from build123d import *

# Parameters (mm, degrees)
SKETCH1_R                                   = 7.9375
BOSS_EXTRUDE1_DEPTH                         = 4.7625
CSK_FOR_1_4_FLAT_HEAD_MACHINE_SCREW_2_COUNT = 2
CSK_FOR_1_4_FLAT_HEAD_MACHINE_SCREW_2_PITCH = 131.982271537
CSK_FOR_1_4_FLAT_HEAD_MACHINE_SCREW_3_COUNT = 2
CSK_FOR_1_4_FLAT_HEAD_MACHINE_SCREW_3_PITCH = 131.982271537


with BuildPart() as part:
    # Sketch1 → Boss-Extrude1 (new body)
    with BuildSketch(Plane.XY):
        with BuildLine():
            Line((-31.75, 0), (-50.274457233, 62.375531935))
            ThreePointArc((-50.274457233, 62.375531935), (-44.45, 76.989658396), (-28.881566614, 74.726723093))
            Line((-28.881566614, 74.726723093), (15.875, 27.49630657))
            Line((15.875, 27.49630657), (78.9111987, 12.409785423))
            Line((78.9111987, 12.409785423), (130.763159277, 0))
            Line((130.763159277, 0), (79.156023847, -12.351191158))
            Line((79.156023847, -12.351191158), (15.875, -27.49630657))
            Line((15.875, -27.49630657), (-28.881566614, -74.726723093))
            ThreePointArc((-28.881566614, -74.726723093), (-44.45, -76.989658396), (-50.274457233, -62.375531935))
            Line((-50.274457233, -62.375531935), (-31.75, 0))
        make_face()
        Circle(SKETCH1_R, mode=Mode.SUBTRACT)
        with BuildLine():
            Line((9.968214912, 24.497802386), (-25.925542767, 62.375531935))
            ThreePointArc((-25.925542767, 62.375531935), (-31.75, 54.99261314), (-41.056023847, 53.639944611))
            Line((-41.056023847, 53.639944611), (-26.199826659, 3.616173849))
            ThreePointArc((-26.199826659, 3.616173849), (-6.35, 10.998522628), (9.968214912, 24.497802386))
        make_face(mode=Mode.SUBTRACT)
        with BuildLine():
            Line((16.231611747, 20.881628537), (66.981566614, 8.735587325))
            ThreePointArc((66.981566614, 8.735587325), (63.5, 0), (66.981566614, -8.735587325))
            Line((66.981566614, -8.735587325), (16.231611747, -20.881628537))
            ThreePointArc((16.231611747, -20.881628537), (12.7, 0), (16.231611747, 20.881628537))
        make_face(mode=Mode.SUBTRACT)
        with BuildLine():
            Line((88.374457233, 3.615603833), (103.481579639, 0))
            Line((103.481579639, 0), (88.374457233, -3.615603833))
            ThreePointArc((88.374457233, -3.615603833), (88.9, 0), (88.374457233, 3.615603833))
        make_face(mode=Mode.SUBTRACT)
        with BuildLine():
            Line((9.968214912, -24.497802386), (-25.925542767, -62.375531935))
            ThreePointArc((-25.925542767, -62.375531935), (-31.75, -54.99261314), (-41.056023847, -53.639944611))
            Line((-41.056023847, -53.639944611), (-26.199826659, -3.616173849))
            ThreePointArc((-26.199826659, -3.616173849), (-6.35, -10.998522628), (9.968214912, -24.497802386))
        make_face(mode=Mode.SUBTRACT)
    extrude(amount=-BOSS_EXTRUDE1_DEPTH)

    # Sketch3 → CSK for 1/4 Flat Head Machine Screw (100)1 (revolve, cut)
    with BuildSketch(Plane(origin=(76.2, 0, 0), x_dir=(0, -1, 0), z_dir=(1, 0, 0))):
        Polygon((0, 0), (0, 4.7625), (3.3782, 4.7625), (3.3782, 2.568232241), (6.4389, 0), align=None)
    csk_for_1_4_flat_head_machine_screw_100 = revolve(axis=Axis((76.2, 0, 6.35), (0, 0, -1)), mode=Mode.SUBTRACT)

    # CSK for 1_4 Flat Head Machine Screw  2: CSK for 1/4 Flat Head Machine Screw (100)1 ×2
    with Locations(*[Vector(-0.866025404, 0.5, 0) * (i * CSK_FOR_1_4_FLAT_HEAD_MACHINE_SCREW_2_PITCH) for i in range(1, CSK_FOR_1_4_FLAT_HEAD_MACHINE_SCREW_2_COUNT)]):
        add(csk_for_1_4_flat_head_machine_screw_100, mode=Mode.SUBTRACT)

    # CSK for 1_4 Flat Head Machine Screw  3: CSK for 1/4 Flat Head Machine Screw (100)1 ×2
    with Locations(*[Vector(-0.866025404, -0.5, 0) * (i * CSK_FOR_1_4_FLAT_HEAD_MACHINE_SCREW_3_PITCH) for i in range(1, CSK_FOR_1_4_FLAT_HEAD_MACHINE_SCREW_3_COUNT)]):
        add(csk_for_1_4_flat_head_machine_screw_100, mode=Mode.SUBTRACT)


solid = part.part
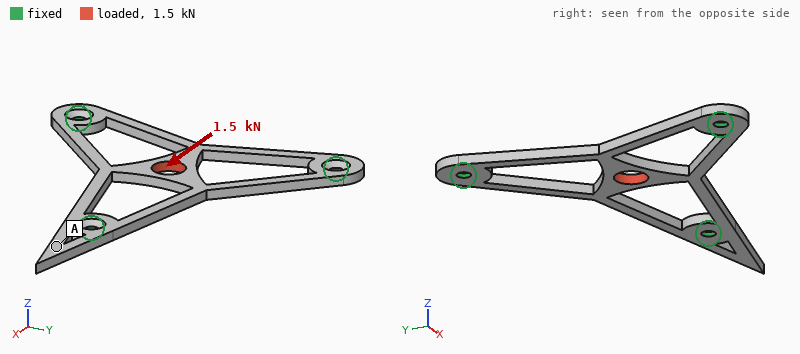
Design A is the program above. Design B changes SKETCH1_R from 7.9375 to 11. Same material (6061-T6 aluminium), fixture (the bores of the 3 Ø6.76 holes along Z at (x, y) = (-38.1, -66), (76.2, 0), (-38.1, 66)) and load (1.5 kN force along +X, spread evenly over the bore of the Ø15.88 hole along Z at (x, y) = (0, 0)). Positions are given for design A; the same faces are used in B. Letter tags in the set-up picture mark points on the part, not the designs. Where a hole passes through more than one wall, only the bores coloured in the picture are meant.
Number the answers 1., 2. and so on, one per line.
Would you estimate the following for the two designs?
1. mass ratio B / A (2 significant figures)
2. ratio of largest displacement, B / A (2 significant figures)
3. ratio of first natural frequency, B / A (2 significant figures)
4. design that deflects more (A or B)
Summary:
1. 0.96
2. 2.0
3. 1.0
4. B
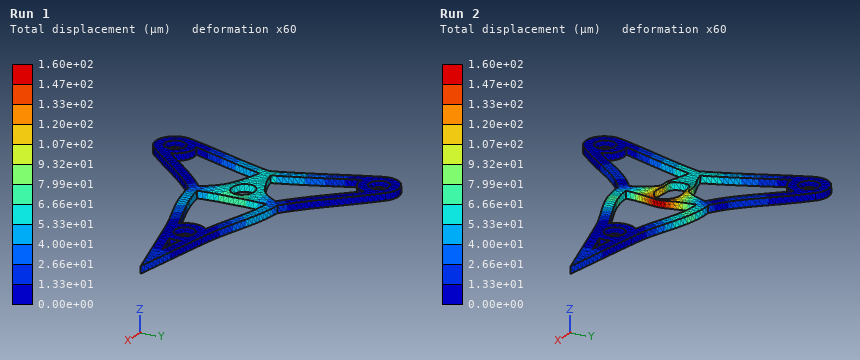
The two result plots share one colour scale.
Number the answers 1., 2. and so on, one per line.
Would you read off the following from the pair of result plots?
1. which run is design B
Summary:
1. Run 2
